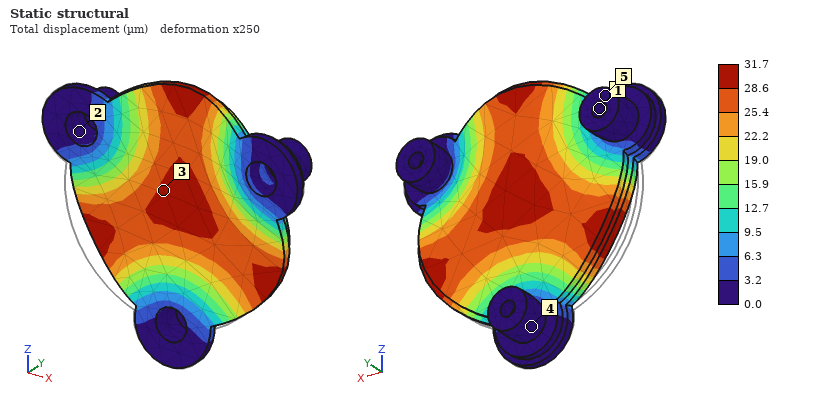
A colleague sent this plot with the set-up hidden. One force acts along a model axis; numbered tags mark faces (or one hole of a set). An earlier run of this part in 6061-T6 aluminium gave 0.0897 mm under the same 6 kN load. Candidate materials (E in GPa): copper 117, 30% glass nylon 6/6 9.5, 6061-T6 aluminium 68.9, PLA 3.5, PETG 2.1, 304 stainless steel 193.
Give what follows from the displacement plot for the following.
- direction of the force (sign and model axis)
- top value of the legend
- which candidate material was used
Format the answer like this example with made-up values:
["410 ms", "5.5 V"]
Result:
["+Y", "31.7 µm", "304 stainless steel"]
